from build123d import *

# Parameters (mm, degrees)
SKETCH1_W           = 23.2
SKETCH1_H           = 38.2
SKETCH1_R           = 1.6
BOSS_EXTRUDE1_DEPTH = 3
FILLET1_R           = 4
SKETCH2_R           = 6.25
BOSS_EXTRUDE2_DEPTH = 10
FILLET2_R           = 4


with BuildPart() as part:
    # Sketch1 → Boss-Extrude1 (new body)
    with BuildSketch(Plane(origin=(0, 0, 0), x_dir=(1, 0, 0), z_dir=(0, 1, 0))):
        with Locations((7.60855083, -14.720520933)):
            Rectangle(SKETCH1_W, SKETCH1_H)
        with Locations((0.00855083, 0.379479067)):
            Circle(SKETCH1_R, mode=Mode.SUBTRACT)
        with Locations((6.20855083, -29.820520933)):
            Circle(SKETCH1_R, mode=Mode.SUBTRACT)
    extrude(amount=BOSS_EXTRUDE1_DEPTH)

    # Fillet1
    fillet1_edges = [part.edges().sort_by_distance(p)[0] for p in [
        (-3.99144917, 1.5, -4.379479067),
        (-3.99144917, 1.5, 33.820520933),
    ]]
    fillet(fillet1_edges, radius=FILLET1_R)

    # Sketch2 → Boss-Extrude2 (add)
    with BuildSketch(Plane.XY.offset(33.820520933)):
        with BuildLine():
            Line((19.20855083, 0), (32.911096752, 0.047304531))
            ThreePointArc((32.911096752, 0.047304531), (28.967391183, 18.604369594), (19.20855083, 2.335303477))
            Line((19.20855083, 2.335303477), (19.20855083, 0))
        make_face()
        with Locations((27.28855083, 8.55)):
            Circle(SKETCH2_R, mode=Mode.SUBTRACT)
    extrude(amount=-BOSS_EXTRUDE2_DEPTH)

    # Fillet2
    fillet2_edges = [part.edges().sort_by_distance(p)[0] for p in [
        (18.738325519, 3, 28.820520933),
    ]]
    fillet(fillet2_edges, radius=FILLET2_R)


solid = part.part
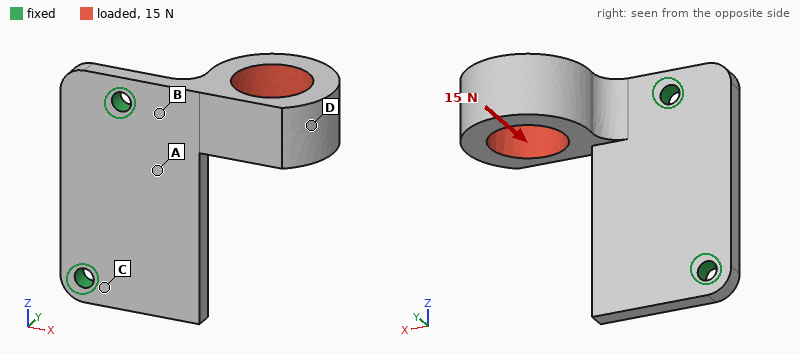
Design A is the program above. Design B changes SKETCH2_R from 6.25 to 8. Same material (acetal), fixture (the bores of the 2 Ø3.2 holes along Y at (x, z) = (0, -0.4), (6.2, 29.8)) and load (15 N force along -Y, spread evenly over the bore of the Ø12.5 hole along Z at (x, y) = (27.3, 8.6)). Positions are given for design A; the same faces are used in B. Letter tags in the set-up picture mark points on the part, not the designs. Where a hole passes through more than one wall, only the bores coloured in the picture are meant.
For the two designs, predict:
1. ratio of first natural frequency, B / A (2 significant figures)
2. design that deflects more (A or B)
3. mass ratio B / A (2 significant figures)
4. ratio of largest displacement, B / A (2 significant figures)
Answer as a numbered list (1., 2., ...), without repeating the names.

1. 1.1
2. B
3. 0.83
4. 1.3
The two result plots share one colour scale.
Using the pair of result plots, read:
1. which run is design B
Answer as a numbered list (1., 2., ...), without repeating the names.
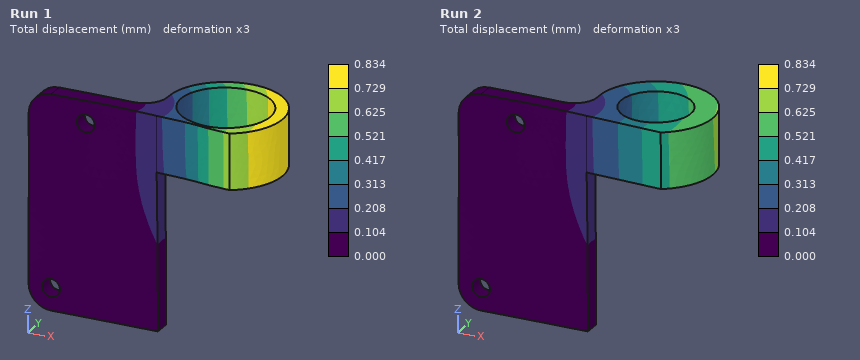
1. Run 1
